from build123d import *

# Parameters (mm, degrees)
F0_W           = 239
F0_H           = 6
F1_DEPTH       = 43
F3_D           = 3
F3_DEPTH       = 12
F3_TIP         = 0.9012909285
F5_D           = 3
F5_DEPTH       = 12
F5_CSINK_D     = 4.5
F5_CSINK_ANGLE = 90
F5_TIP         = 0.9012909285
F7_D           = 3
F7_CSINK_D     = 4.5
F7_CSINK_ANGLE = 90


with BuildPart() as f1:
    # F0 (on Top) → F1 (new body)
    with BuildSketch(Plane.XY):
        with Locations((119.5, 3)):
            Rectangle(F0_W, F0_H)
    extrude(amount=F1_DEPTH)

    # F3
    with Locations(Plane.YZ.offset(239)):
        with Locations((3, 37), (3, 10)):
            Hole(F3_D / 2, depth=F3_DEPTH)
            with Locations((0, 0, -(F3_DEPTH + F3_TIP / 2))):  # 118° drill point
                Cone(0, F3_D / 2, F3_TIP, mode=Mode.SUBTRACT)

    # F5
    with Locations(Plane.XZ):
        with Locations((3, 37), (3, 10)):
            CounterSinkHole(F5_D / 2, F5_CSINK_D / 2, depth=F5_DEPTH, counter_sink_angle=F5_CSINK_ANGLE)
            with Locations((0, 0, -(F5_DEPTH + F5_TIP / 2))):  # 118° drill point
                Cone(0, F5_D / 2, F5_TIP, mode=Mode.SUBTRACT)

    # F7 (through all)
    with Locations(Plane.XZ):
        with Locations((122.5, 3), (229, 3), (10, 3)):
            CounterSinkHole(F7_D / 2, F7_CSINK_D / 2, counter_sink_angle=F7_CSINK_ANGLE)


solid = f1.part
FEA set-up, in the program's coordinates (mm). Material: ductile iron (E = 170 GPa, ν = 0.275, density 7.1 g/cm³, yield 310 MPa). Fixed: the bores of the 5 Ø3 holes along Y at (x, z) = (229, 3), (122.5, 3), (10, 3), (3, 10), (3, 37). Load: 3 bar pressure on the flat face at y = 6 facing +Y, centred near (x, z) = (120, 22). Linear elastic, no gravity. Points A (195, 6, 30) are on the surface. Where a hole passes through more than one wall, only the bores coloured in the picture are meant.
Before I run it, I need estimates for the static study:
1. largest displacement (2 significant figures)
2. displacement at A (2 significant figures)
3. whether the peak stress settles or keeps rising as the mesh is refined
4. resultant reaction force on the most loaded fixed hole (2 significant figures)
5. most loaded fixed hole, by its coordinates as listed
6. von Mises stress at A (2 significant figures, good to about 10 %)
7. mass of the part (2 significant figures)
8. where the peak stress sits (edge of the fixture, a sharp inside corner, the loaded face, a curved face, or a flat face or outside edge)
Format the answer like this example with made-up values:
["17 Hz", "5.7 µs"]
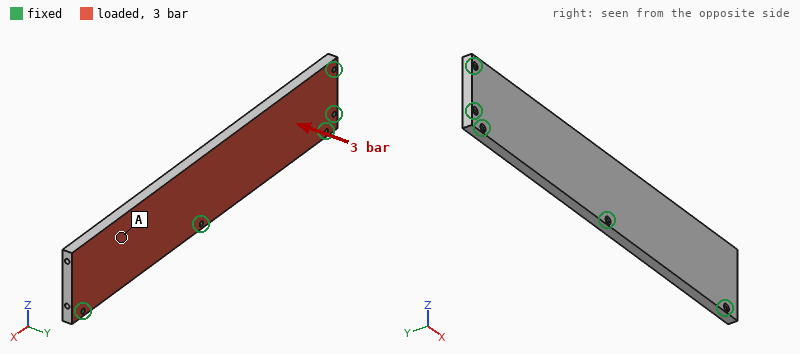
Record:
["0.18 mm", "0.12 mm", "keeps rising", "1.5 kN", "(122.5, 3)", "24 MPa", "430 g", "edge of the fixture"]
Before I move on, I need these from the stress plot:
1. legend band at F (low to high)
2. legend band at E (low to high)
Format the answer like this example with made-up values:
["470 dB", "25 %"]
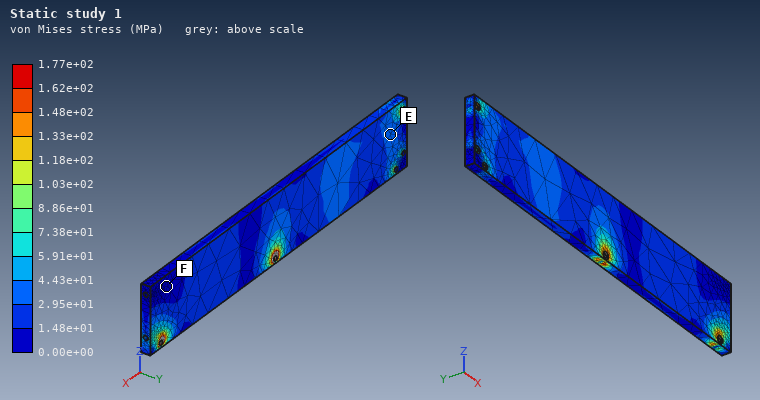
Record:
["0.00e+00 to 1.48e+01 MPa", "2.95e+01 to 4.43e+01 MPa"]
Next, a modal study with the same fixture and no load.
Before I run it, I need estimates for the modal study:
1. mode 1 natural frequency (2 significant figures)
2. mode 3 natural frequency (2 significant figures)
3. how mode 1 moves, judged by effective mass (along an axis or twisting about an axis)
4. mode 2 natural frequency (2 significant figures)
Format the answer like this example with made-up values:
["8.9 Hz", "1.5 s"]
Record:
["1300 Hz", "2800 Hz", "along Y", "1600 Hz"]
